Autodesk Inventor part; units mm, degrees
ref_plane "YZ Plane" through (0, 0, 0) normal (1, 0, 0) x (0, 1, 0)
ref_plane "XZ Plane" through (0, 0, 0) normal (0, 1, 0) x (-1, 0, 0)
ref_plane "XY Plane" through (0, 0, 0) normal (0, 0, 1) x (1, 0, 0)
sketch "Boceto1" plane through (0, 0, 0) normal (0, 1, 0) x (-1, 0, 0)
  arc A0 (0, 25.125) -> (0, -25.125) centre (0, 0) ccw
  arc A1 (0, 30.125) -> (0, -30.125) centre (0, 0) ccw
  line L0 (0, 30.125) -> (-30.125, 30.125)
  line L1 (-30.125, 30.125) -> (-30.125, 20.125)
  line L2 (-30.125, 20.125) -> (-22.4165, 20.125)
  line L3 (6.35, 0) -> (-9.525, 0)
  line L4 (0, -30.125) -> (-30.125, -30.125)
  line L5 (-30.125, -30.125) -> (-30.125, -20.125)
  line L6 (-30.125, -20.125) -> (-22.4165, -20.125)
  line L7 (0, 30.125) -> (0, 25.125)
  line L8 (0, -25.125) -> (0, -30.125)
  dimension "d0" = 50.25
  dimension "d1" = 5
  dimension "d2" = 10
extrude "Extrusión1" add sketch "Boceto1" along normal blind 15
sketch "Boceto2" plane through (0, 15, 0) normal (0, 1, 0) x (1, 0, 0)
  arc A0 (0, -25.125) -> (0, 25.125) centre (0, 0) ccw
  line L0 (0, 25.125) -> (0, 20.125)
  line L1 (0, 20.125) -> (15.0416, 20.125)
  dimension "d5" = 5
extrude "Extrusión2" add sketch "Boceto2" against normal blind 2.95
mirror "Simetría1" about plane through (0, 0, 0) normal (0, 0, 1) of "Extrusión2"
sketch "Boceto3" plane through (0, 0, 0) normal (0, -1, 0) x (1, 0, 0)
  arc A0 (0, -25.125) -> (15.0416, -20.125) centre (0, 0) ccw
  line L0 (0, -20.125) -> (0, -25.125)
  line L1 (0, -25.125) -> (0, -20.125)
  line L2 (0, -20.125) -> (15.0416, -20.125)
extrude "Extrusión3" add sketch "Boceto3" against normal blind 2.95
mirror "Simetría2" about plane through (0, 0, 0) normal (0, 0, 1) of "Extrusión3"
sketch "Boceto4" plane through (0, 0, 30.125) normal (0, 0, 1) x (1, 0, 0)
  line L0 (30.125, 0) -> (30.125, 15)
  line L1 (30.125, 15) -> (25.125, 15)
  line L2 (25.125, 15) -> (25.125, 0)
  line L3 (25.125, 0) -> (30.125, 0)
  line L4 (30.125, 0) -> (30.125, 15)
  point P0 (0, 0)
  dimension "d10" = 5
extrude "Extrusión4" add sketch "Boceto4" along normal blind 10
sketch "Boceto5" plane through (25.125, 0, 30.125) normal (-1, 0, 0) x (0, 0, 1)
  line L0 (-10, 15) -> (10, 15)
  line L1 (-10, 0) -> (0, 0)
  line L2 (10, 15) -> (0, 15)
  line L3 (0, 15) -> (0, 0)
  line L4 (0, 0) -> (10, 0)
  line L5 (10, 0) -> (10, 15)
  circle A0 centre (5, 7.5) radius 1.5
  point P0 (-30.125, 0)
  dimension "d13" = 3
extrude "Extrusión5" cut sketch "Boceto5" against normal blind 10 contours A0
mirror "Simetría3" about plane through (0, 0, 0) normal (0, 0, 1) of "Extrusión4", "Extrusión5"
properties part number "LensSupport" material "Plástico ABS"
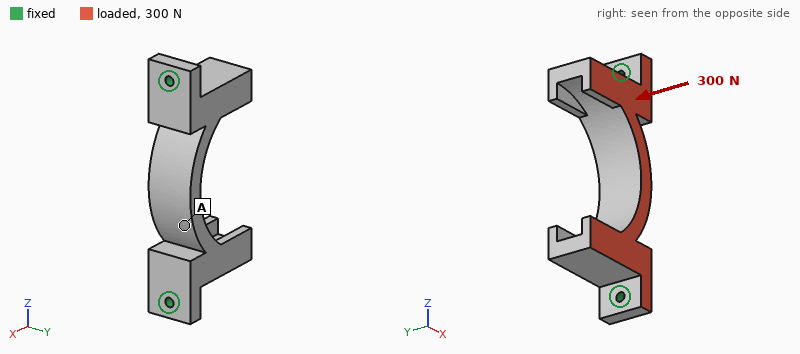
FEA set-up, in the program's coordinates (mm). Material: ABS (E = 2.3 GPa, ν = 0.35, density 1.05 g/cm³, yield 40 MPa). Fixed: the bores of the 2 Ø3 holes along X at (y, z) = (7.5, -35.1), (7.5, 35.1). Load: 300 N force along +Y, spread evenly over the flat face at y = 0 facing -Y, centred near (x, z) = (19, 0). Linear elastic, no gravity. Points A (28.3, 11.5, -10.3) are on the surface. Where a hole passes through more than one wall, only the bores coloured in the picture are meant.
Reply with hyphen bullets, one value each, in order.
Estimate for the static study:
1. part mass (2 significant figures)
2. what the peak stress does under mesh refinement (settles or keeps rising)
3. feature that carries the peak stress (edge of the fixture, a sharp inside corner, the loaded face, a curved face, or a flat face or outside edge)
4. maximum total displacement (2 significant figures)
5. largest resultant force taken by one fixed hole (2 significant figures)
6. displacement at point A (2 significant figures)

- 14 g
- keeps rising
- edge of the fixture
- 0.74 mm
- 150 N
- 0.22 mm
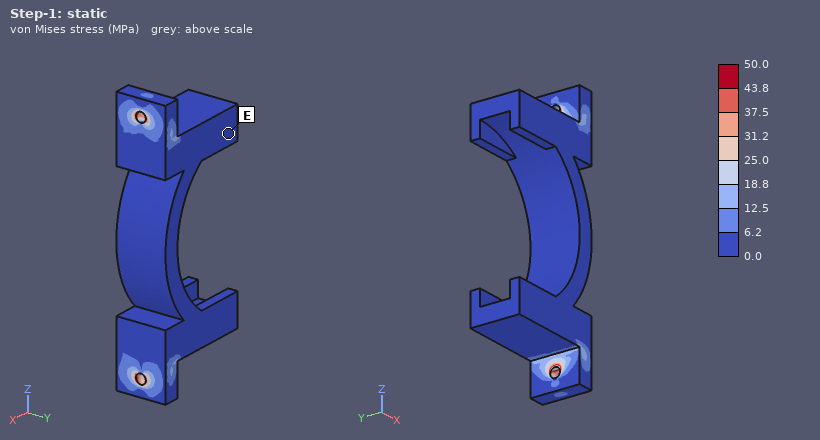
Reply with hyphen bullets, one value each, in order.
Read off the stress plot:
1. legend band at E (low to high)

- 0.0 to 6.2 MPa
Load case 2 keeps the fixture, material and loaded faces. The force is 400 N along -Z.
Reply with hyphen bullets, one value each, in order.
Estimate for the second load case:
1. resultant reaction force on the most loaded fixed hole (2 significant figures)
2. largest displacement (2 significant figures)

- 210 N
- 0.47 mm
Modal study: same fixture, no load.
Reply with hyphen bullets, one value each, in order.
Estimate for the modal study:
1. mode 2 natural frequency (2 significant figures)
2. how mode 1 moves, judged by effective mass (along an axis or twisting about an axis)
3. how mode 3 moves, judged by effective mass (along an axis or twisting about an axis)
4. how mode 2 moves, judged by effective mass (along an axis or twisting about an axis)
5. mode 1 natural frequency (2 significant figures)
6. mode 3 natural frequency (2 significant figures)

- 1200 Hz
- along X
- twisting about X
- along Y
- 980 Hz
- 1400 Hz
